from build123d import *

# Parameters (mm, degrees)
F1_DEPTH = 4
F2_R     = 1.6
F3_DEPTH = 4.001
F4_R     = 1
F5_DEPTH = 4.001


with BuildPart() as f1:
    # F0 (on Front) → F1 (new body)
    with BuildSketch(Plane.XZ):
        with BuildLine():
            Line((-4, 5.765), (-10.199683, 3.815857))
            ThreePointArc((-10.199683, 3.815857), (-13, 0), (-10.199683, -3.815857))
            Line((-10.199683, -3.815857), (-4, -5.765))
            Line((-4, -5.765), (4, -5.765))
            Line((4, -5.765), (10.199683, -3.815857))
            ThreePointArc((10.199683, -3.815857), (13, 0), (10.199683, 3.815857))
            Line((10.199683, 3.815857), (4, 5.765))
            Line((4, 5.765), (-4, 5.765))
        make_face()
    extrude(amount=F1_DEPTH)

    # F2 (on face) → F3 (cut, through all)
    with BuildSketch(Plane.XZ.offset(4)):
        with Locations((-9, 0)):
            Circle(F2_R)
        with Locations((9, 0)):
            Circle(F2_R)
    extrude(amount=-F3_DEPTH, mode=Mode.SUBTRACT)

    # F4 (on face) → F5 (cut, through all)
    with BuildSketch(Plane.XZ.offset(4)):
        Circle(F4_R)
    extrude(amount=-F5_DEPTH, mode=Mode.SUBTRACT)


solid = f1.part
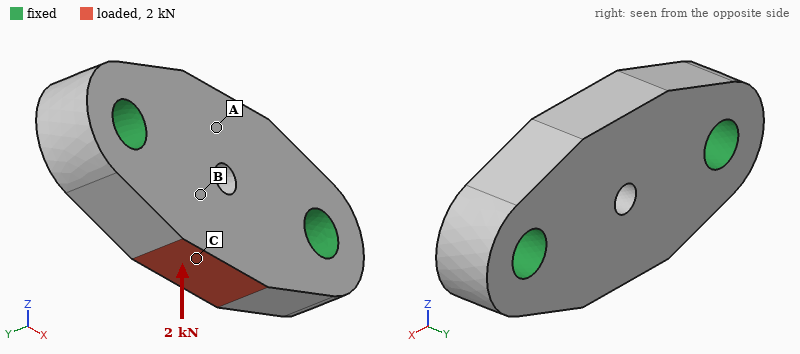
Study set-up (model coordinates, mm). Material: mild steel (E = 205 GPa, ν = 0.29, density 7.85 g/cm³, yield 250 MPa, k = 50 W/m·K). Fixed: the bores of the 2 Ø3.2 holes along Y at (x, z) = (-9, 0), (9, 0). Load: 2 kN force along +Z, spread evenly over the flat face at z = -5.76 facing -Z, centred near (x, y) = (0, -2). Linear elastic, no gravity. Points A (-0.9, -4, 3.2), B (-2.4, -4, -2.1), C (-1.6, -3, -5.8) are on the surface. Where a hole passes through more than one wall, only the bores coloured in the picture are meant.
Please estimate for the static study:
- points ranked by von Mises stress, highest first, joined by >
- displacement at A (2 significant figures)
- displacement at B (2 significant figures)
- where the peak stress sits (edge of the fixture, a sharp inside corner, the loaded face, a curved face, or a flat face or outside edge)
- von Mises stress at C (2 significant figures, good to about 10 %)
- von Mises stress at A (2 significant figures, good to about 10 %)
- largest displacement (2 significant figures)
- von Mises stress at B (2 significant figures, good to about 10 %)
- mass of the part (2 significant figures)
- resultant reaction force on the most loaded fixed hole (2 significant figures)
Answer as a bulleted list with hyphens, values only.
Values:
- C > B > A
- 2.4 µm
- 2.9 µm
- edge of the fixture
- 77 MPa
- 23 MPa
- 4.2 µm
- 52 MPa
- 7.0 g
- 1.0 kN
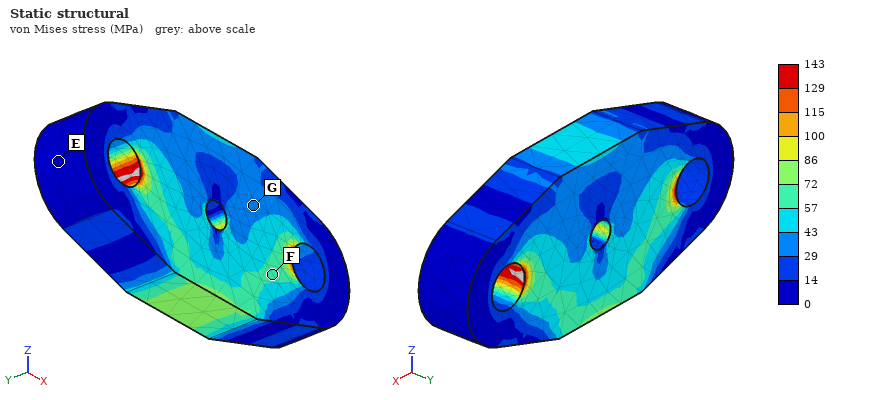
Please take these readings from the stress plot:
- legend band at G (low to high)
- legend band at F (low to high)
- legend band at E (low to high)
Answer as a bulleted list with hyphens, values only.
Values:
- 29 to 43 MPa
- 57 to 72 MPa
- 0 to 14 MPa
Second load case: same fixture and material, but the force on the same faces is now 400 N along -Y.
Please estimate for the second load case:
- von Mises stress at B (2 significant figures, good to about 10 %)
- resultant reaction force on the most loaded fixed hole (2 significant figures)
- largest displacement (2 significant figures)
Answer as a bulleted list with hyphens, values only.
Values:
- 40 MPa
- 200 N
- 5.4 µm
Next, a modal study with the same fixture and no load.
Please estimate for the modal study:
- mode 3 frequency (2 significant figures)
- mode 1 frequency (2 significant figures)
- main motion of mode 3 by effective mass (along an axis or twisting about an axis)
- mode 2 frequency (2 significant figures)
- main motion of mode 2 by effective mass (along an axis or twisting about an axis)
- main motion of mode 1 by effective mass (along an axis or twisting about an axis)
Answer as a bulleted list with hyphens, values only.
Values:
- 72 kHz
- 51 kHz
- along Z
- 53 kHz
- twisting about X
- along Y
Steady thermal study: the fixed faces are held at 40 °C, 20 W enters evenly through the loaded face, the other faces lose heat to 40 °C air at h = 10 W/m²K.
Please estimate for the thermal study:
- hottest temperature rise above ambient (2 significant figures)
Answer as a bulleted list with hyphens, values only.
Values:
- 72 K
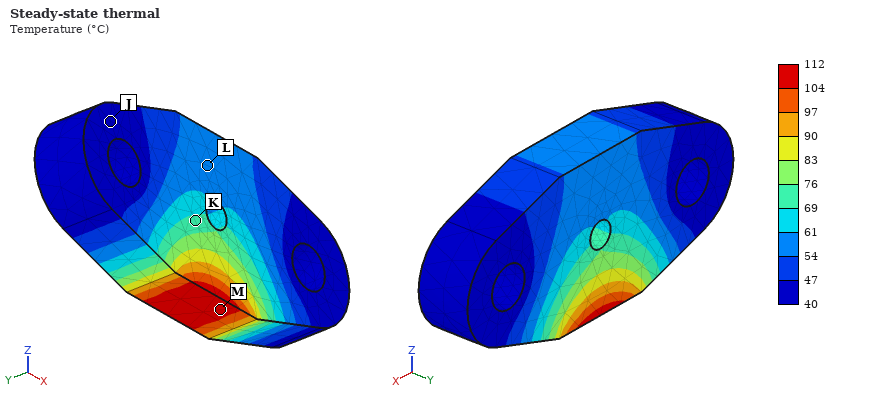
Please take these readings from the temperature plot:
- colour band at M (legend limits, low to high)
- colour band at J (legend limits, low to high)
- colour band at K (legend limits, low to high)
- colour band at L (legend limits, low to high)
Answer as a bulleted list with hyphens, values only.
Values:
- 104 to 112 °C
- 40 to 47 °C
- 69 to 76 °C
- 54 to 61 °C
